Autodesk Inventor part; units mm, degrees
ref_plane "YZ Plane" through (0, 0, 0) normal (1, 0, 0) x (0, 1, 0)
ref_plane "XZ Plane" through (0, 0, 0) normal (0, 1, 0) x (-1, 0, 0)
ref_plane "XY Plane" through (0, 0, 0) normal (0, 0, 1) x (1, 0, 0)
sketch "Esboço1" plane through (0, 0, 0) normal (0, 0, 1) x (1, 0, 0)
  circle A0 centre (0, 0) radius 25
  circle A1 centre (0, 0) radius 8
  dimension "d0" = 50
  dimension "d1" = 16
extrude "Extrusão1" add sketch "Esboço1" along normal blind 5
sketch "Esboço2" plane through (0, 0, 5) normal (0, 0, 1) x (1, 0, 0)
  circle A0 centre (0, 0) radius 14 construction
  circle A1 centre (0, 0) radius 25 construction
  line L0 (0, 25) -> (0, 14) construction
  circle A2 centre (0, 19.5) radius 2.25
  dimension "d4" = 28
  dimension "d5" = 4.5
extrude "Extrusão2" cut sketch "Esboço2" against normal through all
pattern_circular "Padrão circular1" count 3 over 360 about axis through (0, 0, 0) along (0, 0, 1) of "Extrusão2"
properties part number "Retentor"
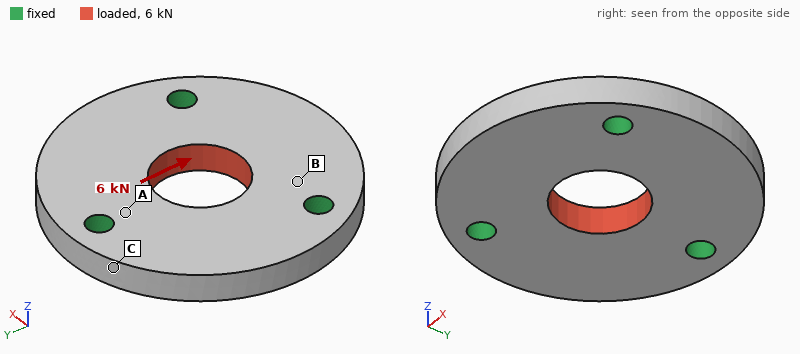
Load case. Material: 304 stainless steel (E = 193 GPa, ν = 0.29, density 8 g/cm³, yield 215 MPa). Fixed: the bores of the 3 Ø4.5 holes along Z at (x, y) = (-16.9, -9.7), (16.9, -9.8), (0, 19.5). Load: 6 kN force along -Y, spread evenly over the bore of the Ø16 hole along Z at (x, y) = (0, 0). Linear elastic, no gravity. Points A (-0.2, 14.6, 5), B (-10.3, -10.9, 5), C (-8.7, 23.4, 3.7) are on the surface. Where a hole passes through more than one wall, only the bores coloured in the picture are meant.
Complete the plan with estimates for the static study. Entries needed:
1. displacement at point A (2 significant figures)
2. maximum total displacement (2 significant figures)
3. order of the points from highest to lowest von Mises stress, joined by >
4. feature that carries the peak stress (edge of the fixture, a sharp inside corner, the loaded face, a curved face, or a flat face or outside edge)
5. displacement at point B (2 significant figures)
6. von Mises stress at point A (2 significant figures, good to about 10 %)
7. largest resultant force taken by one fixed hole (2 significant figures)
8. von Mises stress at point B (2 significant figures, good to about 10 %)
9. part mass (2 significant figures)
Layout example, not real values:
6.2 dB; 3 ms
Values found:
0.59 µm; 3.8 µm; A > B > C; edge of the fixture; 1.7 µm; 42 MPa; 2.1 kN; 24 MPa; 69 g
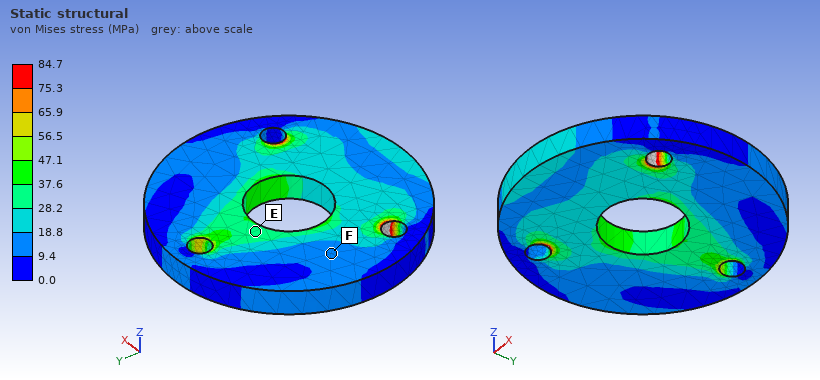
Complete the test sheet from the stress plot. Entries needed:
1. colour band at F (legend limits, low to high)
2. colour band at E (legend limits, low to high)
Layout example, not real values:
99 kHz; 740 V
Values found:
9.4 to 18.8 MPa; 28.2 to 37.6 MPa
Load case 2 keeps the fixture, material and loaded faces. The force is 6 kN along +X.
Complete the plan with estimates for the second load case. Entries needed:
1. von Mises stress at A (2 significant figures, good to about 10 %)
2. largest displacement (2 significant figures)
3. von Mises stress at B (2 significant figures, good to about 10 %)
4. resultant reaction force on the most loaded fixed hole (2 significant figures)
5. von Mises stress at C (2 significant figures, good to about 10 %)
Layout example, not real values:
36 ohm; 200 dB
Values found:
24 MPa; 3.5 µm; 26 MPa; 2.1 kN; 8.4 MPa
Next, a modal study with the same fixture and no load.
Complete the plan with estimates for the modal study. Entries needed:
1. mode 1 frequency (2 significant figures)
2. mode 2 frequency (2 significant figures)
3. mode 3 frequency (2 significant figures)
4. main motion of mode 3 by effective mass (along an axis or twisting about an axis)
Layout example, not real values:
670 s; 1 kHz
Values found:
13 kHz; 13 kHz; 15 kHz; along Z
